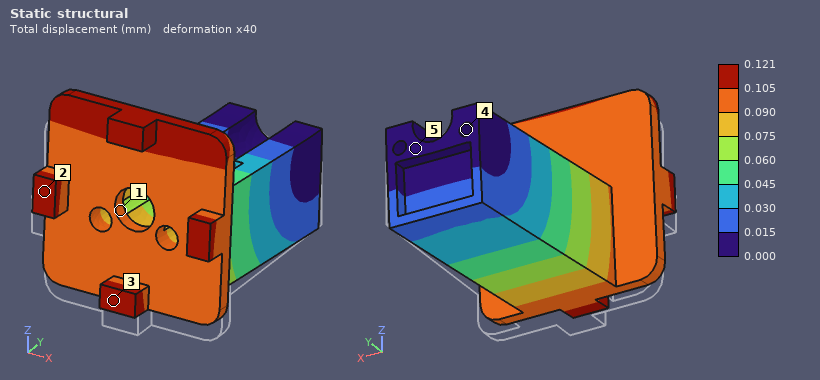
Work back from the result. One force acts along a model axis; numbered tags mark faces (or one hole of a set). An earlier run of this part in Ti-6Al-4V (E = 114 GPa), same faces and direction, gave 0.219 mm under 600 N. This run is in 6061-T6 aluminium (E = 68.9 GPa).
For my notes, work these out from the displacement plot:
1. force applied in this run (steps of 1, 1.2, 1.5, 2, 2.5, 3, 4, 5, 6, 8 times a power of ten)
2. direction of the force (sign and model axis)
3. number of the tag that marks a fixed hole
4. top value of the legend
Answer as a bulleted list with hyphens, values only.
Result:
- 200 N
- +Z
- 4
- 0.121 mm
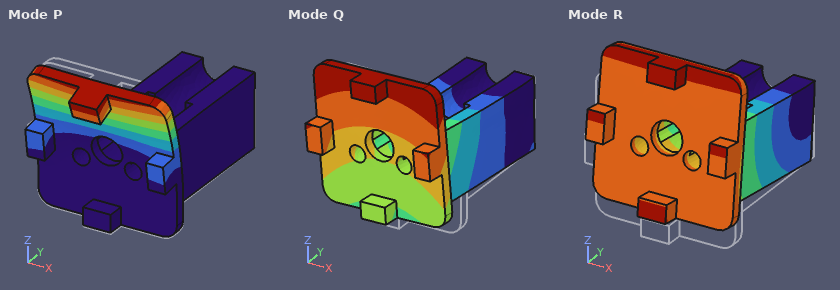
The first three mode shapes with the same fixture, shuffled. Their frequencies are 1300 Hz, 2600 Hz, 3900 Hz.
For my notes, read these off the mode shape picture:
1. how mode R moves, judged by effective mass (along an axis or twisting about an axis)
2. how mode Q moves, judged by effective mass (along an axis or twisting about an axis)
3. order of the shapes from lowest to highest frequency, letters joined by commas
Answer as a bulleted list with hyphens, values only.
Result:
- along Z
- along X
- R, Q, P
